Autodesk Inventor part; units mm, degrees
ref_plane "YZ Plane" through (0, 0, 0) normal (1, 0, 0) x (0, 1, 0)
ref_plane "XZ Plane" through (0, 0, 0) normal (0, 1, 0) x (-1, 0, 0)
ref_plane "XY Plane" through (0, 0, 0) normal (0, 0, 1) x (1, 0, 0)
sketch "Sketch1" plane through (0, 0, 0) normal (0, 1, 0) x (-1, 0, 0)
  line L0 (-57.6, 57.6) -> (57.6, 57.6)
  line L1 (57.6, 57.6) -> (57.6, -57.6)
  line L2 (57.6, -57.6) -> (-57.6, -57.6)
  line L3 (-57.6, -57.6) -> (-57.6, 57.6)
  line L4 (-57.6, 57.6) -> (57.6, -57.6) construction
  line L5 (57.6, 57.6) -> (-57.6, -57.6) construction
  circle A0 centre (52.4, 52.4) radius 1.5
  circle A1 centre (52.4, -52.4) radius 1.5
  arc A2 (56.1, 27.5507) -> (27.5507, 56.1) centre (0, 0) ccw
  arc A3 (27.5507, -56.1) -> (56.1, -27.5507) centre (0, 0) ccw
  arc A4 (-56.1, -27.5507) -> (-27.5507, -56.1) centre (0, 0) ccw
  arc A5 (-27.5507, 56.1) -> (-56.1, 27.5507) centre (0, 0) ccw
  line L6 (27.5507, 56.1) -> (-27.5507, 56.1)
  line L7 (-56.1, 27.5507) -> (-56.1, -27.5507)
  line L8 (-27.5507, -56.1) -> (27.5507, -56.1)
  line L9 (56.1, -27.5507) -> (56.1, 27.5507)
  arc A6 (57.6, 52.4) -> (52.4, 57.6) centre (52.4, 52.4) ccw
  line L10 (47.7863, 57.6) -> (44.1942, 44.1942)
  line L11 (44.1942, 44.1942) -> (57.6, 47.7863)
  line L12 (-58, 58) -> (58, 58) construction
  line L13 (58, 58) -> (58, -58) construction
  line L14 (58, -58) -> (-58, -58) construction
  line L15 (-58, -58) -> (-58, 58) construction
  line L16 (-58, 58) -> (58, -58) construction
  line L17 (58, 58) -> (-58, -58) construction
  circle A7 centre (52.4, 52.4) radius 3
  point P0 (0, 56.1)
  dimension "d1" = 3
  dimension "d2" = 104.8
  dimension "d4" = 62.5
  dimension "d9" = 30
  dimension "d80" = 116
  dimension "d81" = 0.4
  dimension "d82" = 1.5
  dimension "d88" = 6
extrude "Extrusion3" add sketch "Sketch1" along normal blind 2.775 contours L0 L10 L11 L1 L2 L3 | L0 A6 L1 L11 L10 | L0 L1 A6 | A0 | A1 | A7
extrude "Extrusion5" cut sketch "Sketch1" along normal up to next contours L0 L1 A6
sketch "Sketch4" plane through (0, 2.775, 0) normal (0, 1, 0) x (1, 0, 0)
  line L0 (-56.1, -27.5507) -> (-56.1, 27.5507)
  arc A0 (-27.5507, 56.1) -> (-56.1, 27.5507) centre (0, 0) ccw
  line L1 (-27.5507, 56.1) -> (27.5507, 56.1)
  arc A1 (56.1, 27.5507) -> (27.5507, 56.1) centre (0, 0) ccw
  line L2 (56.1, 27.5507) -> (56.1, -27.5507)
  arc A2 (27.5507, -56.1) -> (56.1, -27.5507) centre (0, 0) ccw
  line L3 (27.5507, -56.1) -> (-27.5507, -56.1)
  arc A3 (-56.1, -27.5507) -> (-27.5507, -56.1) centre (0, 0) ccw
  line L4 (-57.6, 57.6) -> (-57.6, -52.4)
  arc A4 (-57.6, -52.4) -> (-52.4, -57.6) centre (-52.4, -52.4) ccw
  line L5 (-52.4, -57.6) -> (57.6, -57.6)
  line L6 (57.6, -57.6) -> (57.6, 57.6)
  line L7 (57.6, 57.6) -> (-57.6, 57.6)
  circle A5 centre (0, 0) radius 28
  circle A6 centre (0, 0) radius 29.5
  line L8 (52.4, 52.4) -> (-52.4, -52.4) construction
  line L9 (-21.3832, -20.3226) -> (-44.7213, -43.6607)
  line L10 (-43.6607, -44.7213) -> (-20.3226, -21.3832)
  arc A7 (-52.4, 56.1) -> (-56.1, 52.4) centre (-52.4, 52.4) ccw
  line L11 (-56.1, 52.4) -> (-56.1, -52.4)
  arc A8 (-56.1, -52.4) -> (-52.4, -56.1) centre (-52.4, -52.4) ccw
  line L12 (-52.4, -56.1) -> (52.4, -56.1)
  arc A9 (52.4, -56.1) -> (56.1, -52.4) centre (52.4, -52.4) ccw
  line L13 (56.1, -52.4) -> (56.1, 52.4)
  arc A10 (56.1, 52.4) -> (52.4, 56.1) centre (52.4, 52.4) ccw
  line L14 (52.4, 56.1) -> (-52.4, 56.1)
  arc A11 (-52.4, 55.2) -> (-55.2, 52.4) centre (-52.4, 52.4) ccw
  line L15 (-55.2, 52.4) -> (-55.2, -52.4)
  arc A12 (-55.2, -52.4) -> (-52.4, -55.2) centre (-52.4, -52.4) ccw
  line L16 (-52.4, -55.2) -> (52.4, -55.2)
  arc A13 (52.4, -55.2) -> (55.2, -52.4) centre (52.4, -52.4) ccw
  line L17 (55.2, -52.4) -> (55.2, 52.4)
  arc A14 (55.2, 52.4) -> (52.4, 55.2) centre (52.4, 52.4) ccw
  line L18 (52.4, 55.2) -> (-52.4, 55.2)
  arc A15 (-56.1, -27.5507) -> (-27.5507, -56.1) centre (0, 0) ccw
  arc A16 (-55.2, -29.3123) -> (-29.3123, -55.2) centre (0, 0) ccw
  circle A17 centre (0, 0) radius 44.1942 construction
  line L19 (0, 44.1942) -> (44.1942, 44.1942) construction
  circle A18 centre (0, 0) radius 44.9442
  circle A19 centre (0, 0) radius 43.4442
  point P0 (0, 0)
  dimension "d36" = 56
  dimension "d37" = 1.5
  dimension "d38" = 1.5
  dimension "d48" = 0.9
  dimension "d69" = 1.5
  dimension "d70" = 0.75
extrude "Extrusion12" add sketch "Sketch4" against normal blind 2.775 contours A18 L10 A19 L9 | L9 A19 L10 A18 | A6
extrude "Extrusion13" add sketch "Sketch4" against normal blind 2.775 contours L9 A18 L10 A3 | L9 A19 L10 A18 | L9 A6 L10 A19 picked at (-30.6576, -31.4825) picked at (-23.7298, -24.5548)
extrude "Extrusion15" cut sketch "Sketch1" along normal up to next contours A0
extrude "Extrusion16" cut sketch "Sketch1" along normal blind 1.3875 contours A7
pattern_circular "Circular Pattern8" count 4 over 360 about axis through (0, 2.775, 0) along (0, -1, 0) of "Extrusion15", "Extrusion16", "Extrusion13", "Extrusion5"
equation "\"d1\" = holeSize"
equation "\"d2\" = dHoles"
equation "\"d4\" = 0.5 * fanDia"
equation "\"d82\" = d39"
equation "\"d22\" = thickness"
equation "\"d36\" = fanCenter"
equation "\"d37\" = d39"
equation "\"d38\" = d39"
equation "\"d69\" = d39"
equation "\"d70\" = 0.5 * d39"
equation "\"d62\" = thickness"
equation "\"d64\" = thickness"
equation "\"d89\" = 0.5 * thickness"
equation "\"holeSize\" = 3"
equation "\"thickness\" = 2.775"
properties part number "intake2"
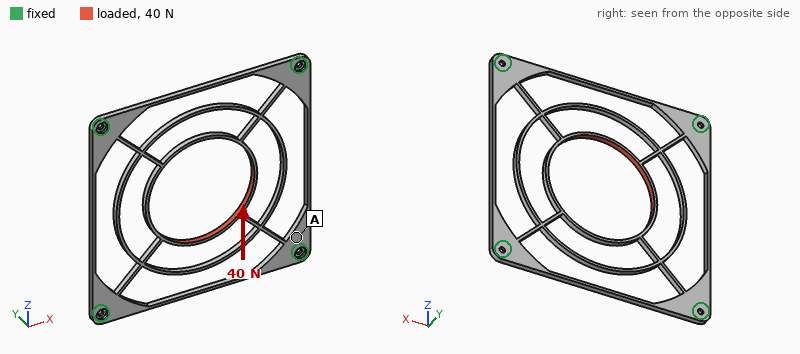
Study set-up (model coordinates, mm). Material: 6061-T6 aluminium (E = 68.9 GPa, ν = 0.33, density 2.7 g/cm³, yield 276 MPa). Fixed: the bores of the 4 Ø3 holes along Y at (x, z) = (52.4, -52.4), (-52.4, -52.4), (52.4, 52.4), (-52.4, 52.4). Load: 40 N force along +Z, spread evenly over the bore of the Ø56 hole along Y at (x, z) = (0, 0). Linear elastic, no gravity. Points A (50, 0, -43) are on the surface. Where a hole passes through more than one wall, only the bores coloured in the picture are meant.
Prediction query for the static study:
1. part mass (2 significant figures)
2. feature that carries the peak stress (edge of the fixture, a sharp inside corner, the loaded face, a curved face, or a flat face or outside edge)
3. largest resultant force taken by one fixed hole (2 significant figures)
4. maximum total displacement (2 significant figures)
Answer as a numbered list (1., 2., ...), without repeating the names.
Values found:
1. 20 g
2. the loaded face
3. 13 N
4. 0.17 mm
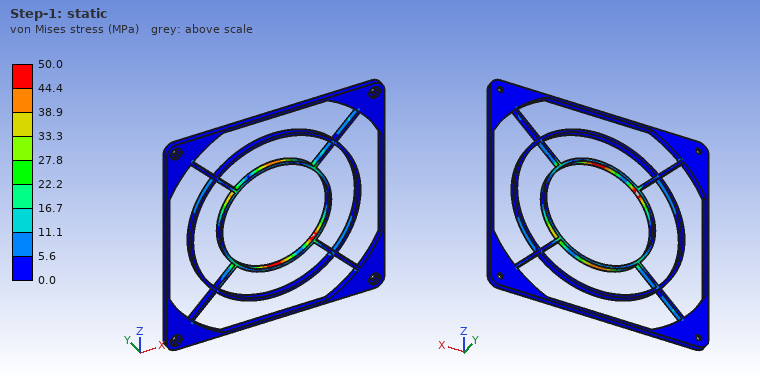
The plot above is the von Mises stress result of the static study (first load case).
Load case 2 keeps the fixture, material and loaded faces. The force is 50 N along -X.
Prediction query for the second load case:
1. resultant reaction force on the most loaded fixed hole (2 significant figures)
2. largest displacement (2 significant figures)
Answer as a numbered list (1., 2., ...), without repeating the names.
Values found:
1. 16 N
2. 0.22 mm
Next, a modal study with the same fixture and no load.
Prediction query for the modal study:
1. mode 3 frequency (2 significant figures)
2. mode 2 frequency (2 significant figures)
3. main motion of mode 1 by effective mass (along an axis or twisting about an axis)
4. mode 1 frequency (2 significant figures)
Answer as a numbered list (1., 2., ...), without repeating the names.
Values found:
1. 1100 Hz
2. 1100 Hz
3. along Y
4. 810 Hz
